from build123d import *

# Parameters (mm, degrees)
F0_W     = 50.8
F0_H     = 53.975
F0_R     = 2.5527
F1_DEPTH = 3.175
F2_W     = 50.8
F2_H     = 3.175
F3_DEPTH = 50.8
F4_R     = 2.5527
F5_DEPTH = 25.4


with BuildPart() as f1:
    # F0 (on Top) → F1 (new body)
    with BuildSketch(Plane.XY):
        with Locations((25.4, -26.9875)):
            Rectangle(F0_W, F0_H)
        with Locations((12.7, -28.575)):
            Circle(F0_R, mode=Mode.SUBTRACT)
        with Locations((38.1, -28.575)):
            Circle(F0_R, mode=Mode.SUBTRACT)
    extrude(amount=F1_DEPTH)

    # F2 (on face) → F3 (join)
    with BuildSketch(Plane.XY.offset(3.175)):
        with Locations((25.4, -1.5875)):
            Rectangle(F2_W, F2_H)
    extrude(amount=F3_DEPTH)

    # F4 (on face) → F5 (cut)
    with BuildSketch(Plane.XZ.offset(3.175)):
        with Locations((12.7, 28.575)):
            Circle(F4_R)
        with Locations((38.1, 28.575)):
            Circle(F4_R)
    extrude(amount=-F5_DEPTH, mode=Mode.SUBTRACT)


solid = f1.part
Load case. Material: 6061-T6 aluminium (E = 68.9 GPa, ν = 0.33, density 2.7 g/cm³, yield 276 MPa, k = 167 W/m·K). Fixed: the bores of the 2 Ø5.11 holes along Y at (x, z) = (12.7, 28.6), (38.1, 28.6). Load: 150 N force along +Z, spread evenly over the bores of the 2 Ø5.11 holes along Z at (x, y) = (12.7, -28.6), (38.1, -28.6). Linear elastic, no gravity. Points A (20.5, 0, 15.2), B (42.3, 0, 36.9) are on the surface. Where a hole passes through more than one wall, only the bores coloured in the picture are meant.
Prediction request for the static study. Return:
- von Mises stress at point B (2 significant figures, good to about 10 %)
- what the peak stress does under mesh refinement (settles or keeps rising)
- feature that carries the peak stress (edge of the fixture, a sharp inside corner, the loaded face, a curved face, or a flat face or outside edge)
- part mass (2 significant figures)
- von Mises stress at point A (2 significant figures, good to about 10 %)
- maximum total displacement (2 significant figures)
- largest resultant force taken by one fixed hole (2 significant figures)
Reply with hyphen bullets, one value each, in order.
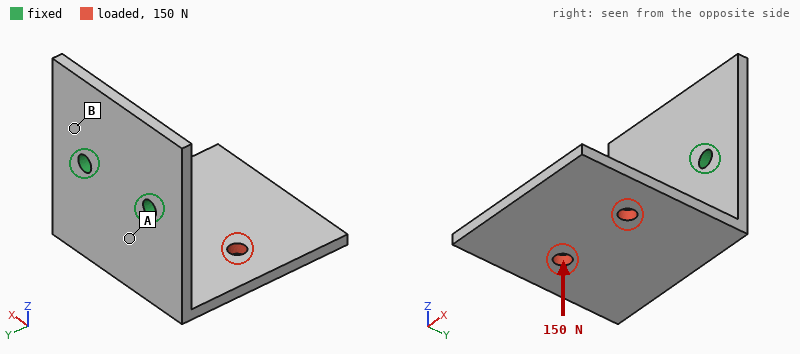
- 6.0 MPa
- keeps rising
- edge of the fixture
- 45 g
- 41 MPa
- 0.79 mm
- 78 N
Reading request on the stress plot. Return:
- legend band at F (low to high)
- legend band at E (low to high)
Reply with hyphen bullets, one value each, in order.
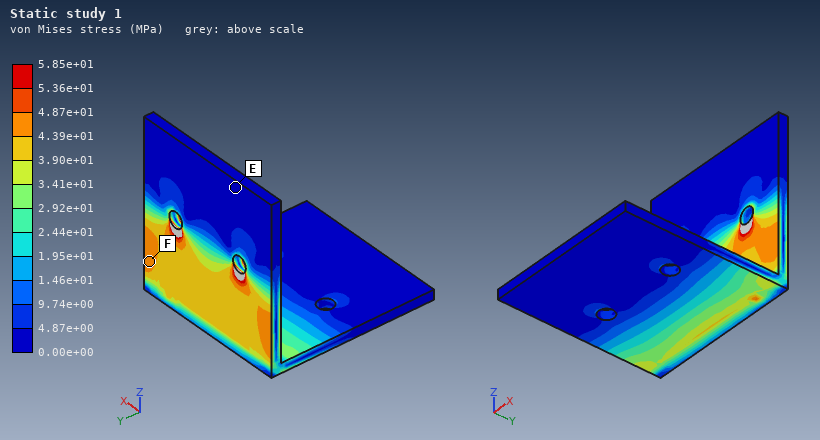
- 4.39e+01 to 4.87e+01 MPa
- 0.00e+00 to 4.87e+00 MPa
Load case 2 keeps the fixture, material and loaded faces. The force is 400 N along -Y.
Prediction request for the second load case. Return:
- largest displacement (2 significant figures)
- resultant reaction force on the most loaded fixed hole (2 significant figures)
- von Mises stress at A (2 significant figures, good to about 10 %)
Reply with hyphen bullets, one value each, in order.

- 0.79 mm
- 200 N
- 57 MPa
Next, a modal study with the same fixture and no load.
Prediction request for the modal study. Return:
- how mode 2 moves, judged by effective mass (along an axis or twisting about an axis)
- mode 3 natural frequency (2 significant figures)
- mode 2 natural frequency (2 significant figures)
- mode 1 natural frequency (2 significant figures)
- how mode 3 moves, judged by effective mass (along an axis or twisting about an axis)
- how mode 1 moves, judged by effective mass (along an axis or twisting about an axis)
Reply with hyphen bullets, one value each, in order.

- along X
- 1800 Hz
- 1000 Hz
- 540 Hz
- along Y
- along Z
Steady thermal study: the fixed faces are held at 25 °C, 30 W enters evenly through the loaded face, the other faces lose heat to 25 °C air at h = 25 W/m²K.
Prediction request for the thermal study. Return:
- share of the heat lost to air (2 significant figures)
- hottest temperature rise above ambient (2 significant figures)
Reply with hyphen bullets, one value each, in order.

- 24 %
- 53 K
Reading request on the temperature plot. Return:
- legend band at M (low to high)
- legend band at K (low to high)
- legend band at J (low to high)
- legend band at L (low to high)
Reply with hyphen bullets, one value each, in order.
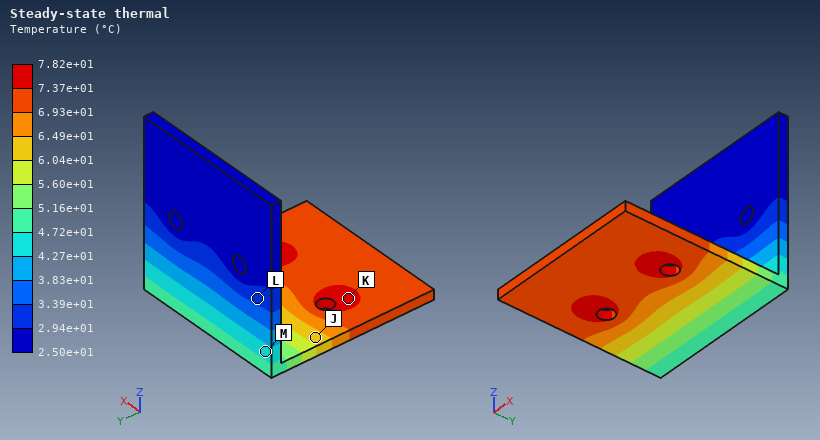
- 4.27e+01 to 4.72e+01 °C
- 7.37e+01 to 7.82e+01 °C
- 6.04e+01 to 6.49e+01 °C
- 2.94e+01 to 3.39e+01 °C
